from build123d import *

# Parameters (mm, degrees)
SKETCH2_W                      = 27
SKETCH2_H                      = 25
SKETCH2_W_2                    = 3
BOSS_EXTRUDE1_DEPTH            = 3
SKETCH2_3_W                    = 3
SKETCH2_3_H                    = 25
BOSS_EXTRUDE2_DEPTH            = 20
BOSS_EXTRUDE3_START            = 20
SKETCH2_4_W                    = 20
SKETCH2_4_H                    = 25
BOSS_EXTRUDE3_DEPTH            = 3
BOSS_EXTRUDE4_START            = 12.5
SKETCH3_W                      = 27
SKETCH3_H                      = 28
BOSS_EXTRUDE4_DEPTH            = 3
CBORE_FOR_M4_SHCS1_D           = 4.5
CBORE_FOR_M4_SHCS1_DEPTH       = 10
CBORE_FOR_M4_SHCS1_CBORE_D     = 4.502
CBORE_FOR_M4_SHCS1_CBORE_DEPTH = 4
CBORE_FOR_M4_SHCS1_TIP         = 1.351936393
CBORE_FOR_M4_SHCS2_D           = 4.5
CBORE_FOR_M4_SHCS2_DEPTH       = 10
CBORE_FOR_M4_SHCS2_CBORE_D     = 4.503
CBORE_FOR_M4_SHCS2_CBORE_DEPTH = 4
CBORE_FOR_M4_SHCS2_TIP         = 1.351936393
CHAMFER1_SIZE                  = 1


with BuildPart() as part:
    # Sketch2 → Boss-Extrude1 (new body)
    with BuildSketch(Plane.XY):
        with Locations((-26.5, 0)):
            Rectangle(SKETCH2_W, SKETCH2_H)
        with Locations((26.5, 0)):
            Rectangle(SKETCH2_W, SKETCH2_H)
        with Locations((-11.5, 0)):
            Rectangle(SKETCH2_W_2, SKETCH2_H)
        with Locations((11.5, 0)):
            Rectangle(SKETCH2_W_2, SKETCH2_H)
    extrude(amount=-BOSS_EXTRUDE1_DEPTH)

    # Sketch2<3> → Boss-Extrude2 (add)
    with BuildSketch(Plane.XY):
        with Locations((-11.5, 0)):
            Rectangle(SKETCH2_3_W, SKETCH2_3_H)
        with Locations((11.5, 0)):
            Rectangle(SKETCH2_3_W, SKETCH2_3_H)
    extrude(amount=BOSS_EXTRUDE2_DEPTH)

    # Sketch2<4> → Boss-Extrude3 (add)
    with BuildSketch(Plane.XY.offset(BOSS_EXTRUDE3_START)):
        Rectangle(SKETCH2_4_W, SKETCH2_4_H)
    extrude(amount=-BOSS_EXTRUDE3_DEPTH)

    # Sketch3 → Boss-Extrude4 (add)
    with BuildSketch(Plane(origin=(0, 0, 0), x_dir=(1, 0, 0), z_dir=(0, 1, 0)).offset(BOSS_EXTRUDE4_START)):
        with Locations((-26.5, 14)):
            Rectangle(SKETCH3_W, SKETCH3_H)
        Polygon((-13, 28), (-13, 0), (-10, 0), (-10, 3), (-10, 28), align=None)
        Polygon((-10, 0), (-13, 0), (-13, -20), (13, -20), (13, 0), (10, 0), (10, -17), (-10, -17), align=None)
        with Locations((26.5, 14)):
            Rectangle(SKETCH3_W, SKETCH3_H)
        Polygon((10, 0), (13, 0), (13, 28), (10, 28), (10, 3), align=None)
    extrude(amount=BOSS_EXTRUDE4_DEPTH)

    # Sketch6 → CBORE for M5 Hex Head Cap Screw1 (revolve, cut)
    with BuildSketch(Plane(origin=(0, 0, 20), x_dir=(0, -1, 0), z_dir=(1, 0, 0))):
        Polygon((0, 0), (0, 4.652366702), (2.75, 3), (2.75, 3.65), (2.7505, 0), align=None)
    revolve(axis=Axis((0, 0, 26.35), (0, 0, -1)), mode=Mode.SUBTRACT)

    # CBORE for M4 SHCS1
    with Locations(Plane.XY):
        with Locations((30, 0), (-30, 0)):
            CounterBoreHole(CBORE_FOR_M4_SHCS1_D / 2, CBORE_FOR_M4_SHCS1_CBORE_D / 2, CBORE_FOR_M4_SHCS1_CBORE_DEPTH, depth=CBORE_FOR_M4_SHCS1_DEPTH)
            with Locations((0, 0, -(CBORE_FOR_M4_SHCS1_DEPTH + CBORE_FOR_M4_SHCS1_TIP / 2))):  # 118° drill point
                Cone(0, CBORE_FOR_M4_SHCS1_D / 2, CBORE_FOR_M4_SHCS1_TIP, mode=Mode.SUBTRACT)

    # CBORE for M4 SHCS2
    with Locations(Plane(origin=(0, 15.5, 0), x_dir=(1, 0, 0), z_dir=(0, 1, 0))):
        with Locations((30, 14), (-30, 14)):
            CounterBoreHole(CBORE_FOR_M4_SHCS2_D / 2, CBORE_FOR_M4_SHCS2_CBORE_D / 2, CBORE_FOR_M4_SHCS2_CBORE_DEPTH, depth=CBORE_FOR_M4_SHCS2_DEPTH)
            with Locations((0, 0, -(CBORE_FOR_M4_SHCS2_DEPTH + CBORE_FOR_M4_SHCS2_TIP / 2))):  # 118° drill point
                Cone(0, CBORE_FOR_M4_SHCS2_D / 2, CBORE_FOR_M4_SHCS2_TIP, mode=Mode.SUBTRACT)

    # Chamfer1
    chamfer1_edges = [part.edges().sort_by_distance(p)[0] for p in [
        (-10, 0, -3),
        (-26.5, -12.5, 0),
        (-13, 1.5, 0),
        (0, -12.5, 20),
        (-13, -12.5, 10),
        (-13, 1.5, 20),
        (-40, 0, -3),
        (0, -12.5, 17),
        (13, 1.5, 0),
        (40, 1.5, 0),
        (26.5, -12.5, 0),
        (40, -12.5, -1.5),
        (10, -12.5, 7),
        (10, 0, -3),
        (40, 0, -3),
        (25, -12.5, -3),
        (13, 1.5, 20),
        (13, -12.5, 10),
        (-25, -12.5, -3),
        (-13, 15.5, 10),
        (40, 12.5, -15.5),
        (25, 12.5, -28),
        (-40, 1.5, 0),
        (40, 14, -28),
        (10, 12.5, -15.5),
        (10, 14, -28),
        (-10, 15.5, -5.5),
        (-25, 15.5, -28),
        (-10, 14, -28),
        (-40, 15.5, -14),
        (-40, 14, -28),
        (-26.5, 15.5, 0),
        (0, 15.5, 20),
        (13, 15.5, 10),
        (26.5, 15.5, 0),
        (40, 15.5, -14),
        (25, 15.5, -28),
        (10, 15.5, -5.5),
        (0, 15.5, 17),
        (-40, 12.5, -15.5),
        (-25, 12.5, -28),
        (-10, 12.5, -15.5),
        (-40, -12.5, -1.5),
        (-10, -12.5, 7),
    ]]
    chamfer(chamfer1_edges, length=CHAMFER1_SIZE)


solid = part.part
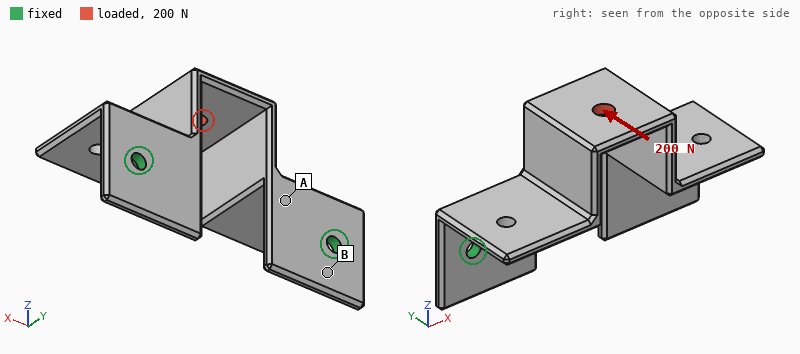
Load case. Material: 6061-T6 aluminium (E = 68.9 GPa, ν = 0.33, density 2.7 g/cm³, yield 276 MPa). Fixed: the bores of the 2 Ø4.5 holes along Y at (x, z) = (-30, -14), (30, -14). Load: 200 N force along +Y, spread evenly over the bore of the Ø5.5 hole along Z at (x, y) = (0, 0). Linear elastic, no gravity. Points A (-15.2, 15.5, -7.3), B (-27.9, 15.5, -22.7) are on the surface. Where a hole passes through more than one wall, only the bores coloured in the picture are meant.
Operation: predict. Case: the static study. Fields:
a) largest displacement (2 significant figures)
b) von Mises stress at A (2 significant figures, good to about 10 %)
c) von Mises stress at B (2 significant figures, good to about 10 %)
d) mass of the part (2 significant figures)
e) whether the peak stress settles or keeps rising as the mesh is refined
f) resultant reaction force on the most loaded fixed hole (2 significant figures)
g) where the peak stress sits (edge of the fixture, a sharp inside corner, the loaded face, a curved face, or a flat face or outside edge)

0.46 mm
55 MPa
14 MPa
37 g
keeps rising
100 N
edge of the fixture
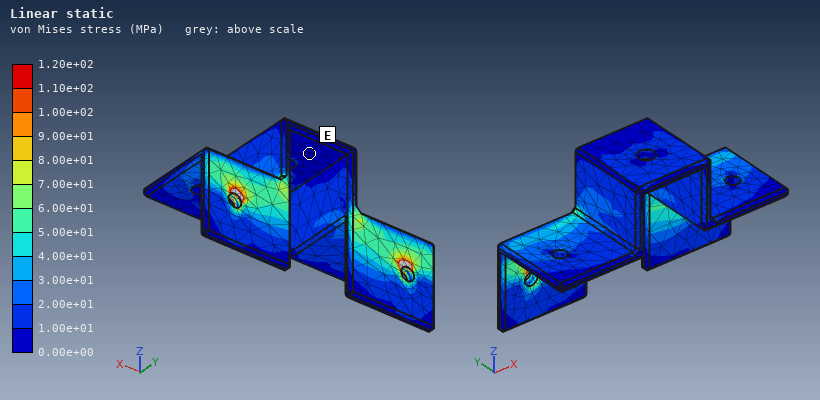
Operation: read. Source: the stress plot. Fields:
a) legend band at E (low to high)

0.00e+00 to 1.00e+01 MPa
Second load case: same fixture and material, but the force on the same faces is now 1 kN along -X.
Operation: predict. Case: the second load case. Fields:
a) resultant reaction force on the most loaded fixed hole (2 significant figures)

710 N
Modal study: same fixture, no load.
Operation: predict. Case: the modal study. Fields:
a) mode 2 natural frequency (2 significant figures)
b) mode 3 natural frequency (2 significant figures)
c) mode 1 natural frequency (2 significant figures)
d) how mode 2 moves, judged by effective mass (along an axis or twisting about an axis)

2800 Hz
3100 Hz
1000 Hz
along X
